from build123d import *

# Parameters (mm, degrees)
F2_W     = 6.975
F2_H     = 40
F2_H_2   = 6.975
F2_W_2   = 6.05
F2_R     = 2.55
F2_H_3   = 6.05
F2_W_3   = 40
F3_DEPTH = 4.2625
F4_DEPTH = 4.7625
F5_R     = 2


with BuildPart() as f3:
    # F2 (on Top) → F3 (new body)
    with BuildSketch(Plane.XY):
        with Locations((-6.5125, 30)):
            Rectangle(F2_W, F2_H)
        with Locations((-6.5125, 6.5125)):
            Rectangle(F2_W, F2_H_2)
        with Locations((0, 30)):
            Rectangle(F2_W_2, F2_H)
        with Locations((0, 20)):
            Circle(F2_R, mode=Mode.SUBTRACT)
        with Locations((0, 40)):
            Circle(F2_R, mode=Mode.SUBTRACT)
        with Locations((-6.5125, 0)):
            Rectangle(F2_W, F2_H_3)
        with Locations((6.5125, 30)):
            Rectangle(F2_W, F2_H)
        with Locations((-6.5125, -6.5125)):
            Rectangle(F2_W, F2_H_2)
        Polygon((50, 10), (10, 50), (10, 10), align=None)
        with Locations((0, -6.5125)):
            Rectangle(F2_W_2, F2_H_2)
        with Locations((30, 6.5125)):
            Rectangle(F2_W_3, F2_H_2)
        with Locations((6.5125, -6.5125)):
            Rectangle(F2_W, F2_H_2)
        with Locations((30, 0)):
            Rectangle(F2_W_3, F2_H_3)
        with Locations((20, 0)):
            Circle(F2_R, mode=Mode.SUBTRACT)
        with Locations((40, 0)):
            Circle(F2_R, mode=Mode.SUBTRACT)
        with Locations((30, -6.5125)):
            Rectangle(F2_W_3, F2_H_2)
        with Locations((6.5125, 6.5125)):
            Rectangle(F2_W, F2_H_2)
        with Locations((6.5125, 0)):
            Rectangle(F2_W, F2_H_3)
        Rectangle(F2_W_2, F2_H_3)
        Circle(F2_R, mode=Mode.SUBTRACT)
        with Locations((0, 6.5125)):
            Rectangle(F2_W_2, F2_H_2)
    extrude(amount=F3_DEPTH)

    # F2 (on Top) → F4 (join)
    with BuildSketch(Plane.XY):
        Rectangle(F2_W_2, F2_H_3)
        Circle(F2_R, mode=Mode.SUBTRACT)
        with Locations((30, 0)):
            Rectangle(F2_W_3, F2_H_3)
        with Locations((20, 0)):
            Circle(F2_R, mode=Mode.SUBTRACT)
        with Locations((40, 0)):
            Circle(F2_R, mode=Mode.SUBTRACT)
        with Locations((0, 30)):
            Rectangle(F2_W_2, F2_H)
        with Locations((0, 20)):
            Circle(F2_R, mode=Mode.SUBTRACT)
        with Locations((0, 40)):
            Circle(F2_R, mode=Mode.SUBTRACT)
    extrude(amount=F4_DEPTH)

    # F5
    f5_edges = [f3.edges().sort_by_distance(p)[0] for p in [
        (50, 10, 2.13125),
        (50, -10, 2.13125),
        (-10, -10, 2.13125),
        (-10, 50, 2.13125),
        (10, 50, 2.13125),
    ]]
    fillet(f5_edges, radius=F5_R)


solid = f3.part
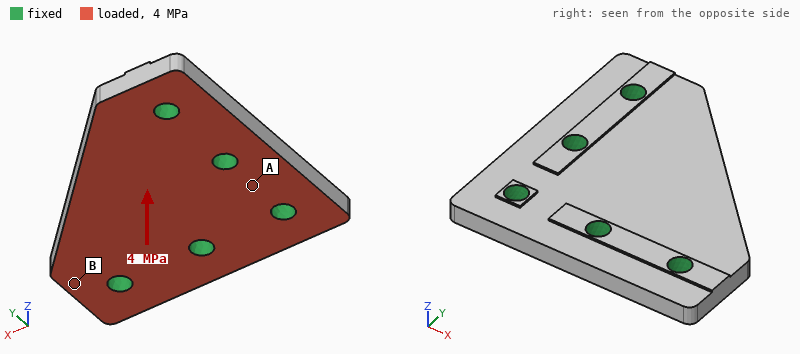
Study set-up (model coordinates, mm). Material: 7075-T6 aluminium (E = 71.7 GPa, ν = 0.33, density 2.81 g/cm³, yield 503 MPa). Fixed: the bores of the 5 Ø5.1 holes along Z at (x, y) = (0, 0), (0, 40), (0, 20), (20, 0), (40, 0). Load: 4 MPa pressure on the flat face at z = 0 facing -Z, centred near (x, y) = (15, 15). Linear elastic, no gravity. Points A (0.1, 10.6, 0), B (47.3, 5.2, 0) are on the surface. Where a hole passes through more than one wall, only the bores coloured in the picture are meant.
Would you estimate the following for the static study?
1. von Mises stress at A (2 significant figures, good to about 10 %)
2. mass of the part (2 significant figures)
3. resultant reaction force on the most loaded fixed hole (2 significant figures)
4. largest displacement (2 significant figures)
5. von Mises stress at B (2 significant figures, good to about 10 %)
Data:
37 MPa
33 g
2.5 kN
0.23 mm
110 MPa
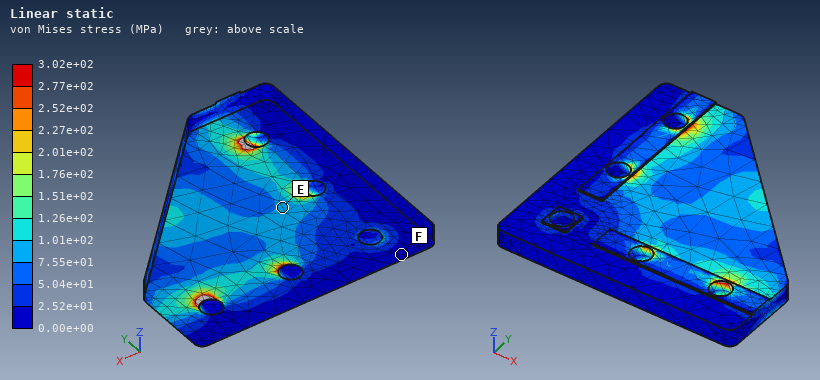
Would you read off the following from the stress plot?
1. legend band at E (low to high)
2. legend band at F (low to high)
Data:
7.55e+01 to 1.01e+02 MPa
0.00e+00 to 2.52e+01 MPa
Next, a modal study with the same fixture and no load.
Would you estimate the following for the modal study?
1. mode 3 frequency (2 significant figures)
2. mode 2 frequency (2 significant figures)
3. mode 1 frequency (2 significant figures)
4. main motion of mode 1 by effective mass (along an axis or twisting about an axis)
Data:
23 kHz
17 kHz
8300 Hz
along Z
